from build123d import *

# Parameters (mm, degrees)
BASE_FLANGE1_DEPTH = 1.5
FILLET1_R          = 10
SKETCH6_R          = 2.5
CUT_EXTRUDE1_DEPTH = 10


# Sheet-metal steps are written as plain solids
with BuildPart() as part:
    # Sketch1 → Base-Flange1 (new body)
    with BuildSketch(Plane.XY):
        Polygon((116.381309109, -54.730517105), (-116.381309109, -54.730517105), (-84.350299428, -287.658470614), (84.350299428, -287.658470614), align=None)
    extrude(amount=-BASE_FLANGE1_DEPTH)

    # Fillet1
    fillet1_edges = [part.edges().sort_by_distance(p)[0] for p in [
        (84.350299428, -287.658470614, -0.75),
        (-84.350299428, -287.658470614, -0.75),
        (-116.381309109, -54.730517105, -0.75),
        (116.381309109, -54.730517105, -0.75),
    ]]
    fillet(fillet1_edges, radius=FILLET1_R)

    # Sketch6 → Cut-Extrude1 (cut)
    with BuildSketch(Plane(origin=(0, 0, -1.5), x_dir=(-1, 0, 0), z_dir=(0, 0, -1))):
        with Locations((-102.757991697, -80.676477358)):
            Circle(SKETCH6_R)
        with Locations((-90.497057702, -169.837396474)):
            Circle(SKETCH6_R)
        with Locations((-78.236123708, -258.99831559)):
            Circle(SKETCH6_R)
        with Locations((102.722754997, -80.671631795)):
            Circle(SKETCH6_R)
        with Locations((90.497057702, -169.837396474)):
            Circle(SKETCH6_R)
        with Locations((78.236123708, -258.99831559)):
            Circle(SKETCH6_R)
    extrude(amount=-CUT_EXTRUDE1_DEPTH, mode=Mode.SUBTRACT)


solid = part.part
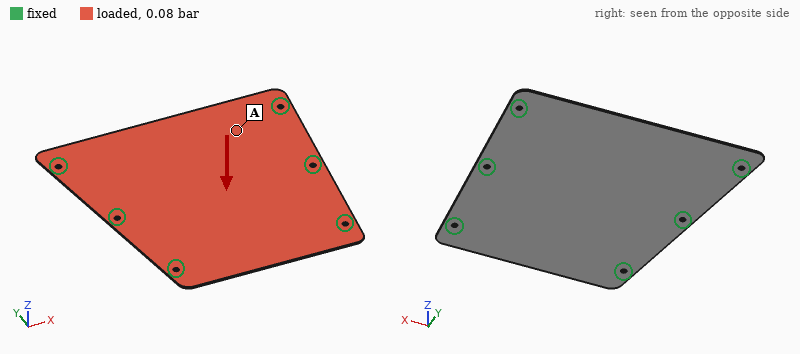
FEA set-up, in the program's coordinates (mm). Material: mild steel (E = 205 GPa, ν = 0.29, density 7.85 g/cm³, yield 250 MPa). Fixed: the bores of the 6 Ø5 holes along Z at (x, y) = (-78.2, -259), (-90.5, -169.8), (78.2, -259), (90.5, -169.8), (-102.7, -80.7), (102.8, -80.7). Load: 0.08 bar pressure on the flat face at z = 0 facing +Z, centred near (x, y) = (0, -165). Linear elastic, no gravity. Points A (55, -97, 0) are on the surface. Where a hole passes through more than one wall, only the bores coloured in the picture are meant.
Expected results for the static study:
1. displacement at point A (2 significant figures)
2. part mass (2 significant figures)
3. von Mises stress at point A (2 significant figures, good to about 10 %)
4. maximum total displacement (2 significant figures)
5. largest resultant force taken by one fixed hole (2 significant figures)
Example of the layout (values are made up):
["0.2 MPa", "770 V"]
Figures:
["0.38 mm", "550 g", "13 MPa", "0.78 mm", "73 N"]
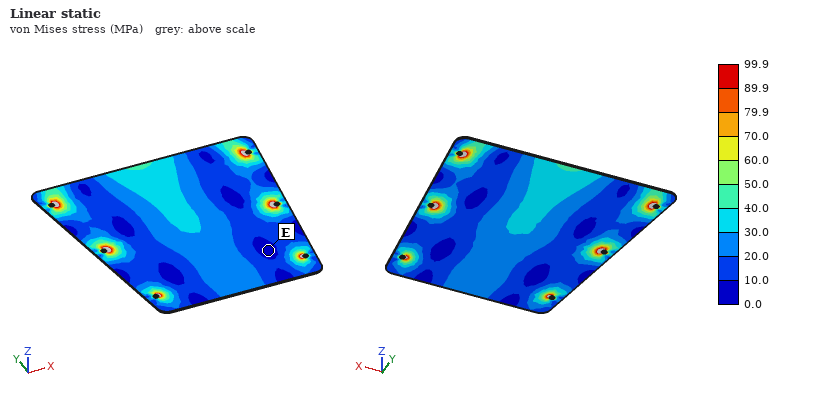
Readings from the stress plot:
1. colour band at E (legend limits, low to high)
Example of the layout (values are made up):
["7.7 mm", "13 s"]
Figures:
["0.0 to 10.0 MPa"]
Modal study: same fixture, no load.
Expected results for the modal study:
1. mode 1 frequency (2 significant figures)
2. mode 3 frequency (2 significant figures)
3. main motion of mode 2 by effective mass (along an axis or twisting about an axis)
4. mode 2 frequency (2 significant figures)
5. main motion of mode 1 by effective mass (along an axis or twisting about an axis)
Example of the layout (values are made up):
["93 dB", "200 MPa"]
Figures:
["190 Hz", "370 Hz", "along Z", "280 Hz", "along Z"]
